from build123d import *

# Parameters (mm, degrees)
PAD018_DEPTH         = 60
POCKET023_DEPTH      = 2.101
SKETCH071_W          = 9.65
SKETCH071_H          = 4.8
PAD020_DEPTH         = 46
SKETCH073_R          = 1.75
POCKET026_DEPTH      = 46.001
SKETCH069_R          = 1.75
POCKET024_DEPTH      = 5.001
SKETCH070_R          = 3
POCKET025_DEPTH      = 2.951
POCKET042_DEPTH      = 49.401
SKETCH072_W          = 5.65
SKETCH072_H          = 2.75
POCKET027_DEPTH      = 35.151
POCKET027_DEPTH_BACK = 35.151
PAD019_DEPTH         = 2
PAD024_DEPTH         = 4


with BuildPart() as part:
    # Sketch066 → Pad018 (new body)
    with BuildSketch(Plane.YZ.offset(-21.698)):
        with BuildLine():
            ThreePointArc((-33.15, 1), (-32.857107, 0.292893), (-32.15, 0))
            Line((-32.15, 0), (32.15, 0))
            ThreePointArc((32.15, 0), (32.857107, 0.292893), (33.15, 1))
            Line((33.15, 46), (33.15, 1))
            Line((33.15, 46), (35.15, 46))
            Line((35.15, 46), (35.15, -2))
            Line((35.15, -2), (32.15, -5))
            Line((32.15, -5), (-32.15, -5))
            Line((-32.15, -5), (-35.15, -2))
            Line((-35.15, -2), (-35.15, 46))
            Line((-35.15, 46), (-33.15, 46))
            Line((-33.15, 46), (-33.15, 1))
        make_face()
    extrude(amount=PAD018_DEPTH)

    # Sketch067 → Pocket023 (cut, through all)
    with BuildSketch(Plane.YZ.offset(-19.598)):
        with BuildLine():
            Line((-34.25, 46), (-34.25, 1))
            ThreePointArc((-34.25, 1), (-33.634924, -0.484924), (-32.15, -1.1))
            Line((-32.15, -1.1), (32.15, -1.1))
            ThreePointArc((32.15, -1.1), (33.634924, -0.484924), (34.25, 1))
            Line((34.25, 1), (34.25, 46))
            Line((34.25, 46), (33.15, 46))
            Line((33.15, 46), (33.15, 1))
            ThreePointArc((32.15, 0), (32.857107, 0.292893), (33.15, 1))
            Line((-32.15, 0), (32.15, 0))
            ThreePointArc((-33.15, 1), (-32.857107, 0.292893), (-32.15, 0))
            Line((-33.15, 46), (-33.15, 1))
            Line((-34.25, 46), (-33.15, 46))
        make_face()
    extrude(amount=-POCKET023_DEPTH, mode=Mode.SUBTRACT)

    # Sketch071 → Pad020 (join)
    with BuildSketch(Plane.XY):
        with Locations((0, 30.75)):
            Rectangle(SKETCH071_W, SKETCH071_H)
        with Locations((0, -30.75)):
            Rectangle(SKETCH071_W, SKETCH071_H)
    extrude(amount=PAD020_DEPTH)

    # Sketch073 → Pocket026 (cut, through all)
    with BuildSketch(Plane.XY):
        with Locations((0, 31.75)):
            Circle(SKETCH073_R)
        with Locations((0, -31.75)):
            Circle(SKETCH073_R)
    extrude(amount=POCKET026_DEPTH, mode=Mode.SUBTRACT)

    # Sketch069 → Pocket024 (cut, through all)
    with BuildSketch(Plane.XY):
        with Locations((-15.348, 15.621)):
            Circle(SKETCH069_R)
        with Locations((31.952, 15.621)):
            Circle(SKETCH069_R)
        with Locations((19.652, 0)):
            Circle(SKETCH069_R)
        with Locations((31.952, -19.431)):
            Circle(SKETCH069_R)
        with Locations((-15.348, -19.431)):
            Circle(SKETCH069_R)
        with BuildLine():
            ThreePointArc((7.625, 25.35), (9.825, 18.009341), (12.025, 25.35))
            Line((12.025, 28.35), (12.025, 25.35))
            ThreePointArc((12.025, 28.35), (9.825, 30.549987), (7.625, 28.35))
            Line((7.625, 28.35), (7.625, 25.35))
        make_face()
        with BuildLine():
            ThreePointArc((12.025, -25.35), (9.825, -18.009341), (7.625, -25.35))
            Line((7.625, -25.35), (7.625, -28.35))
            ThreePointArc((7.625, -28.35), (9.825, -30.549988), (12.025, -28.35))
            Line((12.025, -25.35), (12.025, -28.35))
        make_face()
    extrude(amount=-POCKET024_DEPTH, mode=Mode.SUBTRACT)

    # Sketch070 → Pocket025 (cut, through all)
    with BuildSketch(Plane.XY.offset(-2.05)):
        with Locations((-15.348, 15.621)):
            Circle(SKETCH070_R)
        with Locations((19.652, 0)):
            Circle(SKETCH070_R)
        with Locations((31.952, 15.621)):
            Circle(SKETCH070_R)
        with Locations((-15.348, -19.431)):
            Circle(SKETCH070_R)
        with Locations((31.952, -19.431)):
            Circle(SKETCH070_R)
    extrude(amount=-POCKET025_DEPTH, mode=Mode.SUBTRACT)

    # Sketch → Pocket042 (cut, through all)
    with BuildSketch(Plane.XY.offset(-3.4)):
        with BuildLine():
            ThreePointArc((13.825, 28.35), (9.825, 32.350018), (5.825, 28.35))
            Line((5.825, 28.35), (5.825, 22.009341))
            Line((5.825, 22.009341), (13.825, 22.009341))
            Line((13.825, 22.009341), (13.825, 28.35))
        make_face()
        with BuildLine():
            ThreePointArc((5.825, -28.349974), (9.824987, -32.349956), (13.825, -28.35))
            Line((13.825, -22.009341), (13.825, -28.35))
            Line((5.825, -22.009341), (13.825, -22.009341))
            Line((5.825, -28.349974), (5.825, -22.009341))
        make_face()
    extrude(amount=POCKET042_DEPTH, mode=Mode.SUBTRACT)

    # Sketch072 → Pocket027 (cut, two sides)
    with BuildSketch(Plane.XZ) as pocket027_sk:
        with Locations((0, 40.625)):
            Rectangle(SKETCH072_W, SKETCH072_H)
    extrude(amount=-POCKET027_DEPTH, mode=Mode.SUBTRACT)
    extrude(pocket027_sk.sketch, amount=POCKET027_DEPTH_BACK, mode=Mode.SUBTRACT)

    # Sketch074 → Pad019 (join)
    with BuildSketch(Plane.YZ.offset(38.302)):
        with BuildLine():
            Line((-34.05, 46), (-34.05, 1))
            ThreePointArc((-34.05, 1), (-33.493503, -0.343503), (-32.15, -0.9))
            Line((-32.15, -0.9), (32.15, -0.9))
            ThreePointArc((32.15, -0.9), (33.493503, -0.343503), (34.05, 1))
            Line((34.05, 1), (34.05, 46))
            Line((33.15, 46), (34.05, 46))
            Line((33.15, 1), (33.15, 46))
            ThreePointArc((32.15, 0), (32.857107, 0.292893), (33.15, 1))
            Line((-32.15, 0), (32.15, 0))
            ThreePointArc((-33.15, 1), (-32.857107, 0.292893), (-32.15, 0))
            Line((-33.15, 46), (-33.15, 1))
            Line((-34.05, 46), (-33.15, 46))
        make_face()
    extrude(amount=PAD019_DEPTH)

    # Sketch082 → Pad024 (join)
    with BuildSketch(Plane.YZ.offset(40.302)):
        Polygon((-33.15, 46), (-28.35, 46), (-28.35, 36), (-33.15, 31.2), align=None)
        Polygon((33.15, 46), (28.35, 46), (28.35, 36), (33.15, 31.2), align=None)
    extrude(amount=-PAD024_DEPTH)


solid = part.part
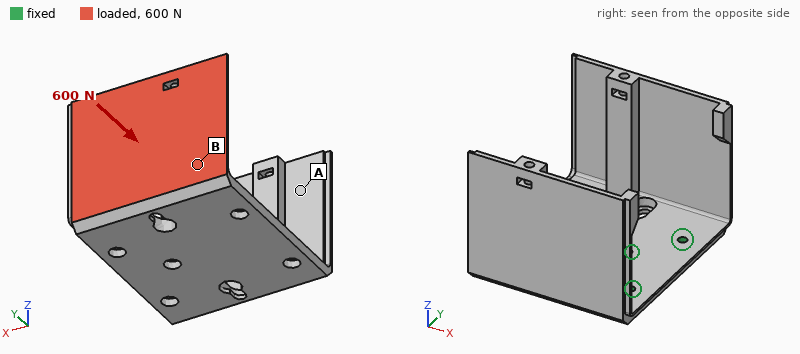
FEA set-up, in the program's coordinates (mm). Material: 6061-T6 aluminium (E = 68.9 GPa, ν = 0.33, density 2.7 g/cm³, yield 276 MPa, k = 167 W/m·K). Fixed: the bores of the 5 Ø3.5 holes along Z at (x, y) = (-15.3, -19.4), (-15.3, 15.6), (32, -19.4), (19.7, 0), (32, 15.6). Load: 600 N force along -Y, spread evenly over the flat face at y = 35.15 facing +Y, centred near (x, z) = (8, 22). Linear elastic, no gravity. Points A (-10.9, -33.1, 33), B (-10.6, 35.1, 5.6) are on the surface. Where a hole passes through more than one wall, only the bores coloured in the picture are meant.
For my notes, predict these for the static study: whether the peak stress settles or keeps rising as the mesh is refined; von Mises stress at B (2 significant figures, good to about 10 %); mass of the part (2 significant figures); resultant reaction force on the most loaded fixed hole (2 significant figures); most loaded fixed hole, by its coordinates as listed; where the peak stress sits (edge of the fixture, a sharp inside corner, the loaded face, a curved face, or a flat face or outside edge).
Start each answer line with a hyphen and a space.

- keeps rising
- 45 MPa
- 91 g
- 760 N
- (-15.3, 15.6)
- edge of the fixture
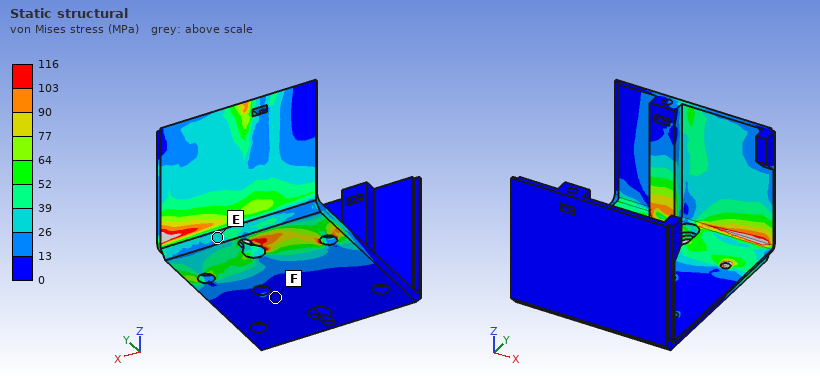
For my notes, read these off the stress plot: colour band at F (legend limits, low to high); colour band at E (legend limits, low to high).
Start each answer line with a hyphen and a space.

- 0 to 13 MPa
- 26 to 39 MPa
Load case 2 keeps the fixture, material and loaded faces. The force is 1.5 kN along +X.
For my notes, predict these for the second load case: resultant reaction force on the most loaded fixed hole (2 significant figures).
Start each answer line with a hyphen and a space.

- 1.3 kN
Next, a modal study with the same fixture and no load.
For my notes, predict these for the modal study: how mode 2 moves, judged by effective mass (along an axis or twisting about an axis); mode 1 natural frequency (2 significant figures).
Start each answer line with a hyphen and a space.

- along Y
- 1100 Hz
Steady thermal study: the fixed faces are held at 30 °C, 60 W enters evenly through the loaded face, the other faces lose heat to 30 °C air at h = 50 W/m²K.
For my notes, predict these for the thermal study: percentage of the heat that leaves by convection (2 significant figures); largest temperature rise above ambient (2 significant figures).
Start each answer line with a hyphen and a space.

- 26 %
- 69 K
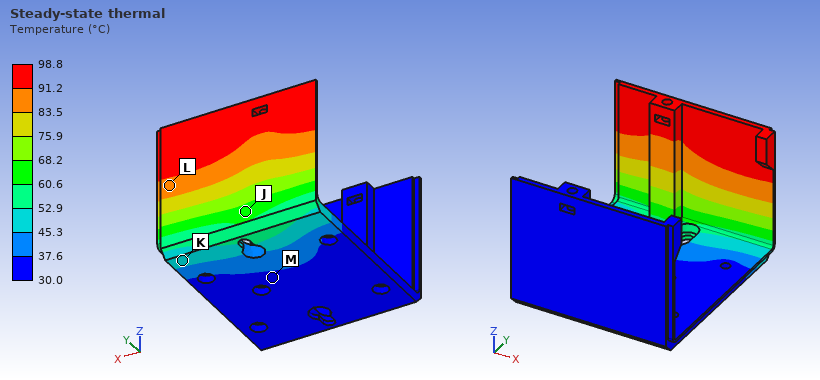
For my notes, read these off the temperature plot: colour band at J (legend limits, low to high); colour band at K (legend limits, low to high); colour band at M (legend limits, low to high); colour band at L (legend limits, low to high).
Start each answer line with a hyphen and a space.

- 60.6 to 68.2 °C
- 45.3 to 52.9 °C
- 30.0 to 37.6 °C
- 83.5 to 91.2 °C
